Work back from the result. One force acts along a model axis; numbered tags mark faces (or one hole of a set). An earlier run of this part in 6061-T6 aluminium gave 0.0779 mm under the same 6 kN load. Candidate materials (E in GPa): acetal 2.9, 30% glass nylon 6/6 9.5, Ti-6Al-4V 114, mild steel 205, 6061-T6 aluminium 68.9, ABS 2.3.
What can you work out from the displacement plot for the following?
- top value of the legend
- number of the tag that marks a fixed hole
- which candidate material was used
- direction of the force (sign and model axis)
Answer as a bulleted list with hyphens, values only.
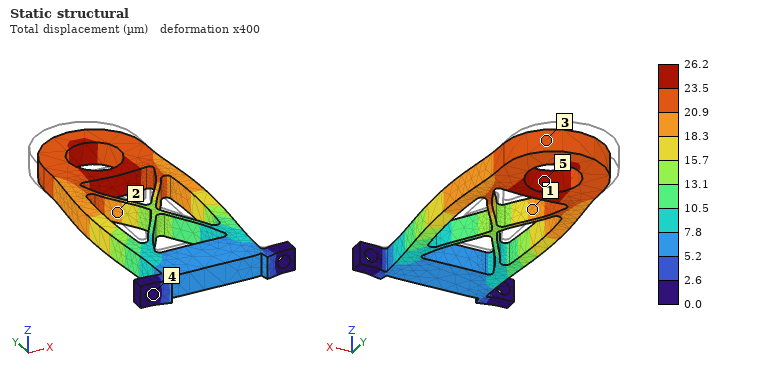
- 26.2 µm
- 4
- mild steel
- -Y
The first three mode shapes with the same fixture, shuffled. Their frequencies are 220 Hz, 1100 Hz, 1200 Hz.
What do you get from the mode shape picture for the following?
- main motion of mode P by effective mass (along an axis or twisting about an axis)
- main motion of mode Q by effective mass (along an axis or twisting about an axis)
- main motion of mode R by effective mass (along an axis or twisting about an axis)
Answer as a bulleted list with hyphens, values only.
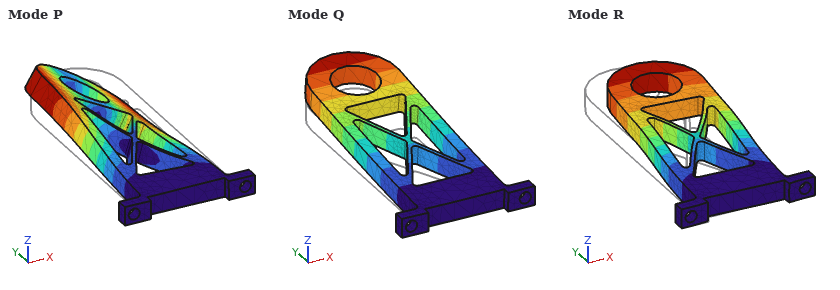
- twisting about Y
- along Z
- along X
